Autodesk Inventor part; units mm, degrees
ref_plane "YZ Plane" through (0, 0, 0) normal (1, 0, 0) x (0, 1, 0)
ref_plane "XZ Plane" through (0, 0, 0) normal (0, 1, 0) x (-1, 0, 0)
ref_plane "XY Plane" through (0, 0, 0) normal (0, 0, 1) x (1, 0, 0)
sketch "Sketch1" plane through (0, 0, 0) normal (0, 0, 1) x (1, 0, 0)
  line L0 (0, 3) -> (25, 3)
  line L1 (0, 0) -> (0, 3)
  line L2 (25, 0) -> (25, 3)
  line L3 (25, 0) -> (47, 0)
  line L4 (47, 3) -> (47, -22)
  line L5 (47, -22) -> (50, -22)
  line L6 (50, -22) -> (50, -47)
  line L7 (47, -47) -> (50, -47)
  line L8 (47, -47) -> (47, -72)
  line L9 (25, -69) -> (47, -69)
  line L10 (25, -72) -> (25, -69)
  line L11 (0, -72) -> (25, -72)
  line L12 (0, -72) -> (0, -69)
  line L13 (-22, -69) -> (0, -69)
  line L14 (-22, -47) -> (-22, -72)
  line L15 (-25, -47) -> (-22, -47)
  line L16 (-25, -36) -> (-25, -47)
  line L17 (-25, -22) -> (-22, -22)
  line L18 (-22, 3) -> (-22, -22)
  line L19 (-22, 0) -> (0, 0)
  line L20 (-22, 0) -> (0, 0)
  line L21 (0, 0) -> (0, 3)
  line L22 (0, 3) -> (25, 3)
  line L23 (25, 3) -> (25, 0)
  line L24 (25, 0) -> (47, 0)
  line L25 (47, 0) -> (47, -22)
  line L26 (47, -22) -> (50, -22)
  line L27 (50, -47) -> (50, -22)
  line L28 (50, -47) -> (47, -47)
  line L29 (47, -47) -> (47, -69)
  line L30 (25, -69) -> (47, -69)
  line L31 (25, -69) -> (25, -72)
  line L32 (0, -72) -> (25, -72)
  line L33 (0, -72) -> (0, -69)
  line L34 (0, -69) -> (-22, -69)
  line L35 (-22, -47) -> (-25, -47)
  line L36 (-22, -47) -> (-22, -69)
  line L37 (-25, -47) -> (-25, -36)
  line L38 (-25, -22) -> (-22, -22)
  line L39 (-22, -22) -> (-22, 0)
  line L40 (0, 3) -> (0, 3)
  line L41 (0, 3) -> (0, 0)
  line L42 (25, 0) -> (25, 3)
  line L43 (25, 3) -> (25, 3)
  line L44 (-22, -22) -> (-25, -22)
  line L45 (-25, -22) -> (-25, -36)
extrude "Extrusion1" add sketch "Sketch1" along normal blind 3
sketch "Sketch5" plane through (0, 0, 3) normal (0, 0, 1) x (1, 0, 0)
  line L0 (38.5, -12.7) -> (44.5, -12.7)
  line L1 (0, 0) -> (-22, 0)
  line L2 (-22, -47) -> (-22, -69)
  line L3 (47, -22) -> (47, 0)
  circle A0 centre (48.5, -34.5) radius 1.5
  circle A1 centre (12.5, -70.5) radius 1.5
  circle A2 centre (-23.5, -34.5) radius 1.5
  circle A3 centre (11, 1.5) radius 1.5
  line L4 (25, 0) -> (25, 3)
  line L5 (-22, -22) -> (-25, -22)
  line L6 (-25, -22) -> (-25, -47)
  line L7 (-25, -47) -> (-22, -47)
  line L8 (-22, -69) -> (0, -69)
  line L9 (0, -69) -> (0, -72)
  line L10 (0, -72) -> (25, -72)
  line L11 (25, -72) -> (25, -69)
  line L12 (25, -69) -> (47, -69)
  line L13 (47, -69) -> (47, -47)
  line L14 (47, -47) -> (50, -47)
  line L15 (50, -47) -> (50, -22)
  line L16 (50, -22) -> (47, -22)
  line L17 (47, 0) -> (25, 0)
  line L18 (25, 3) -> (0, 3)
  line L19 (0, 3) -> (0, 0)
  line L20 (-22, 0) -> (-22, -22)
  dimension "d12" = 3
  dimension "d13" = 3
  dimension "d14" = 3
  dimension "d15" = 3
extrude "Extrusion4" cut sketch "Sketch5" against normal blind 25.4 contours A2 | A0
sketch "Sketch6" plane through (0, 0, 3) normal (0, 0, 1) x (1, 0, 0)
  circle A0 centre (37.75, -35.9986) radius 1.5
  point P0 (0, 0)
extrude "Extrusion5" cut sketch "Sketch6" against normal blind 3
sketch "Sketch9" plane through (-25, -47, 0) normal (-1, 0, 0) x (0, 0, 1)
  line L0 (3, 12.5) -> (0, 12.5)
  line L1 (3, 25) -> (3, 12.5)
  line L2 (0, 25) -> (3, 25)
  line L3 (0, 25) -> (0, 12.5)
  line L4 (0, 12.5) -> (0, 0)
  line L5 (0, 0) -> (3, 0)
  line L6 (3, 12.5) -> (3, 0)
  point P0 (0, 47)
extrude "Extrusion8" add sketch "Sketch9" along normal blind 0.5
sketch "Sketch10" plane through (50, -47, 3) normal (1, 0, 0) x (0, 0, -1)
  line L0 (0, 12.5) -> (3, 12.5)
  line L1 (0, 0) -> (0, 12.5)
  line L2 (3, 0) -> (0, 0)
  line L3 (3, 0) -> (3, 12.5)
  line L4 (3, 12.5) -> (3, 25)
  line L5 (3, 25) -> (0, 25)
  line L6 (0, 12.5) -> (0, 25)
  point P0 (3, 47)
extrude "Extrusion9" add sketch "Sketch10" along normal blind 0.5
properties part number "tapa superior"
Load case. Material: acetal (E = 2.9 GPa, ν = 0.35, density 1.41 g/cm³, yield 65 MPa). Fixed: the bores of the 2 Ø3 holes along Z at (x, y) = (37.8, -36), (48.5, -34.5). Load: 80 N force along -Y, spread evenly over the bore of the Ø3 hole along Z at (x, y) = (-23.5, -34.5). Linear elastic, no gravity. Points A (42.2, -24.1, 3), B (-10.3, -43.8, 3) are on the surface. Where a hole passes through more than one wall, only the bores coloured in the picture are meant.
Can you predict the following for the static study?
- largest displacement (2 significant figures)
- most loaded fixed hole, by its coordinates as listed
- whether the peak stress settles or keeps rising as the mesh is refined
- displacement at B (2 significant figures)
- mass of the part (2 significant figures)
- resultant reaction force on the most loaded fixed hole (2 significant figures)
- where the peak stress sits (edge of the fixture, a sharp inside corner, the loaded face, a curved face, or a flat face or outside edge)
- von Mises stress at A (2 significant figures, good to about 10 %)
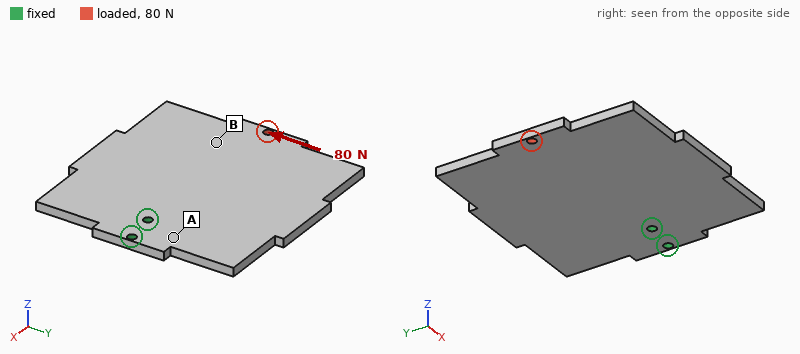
0.58 mm
(37.8, -36)
keeps rising
0.42 mm
21 g
460 N
edge of the fixture
5.3 MPa
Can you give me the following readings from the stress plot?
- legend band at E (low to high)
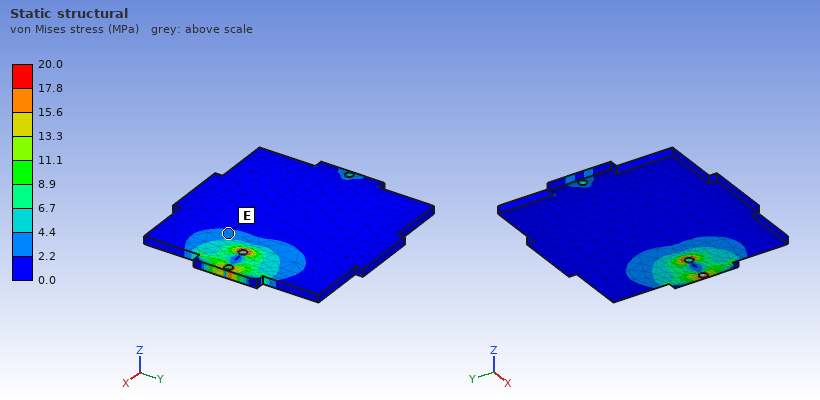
2.2 to 4.4 MPa
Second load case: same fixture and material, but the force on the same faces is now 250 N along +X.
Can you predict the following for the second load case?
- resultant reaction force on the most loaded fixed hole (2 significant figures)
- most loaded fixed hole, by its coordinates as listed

180 N
(37.8, -36)
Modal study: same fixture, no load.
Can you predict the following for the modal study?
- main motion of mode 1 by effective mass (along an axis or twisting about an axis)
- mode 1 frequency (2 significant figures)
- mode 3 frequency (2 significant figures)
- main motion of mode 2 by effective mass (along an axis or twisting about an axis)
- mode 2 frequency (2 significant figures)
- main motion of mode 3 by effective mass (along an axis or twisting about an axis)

along Z
150 Hz
600 Hz
twisting about X
230 Hz
along Z
